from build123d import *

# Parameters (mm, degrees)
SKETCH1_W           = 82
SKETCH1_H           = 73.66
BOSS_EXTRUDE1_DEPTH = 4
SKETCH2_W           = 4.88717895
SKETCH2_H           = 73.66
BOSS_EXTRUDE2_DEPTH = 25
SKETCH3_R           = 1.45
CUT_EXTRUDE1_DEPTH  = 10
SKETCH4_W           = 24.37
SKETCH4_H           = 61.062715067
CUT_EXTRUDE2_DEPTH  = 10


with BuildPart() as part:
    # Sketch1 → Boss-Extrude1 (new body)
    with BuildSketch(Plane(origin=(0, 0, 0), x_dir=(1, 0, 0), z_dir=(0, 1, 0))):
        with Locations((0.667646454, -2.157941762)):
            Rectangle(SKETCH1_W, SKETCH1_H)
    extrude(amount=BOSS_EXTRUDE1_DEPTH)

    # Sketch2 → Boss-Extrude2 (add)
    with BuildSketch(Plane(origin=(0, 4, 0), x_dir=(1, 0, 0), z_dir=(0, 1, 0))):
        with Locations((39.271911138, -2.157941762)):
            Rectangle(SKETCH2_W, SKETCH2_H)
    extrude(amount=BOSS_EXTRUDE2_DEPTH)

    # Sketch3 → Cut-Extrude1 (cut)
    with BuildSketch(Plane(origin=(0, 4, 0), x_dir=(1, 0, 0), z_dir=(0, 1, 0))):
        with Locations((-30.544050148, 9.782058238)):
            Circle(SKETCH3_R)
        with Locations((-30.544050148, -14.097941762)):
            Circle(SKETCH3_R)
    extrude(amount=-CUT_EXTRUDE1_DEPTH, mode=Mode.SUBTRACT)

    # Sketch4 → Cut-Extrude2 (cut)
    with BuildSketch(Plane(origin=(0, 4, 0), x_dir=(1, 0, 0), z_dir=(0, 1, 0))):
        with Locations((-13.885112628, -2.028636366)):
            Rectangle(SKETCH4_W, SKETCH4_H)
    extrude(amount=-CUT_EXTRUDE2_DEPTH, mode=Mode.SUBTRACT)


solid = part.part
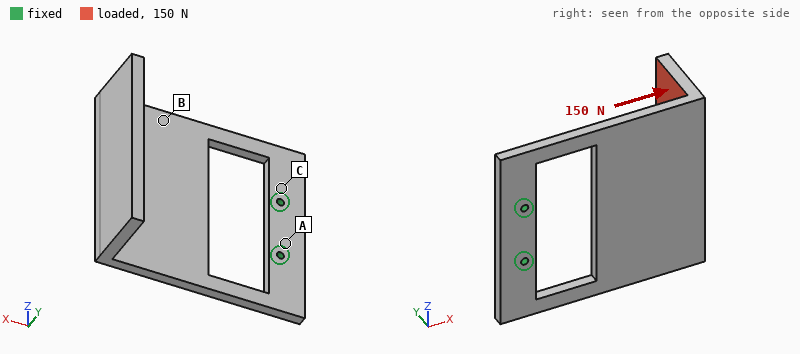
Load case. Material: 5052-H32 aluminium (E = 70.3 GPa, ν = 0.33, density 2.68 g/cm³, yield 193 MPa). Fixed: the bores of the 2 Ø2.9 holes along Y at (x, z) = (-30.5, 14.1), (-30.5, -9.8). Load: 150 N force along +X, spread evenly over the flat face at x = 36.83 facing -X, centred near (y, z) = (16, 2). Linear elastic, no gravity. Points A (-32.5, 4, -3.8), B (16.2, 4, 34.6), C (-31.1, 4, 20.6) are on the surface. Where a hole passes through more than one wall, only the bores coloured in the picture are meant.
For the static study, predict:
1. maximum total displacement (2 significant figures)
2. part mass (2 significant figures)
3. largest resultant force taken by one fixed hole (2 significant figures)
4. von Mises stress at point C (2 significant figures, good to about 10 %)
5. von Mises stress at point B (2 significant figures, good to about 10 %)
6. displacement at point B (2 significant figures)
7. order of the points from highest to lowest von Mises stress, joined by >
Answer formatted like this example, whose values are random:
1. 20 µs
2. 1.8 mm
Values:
1. 1.3 mm
2. 73 g
3. 120 N
4. 32 MPa
5. 16 MPa
6. 0.61 mm
7. C > B > A
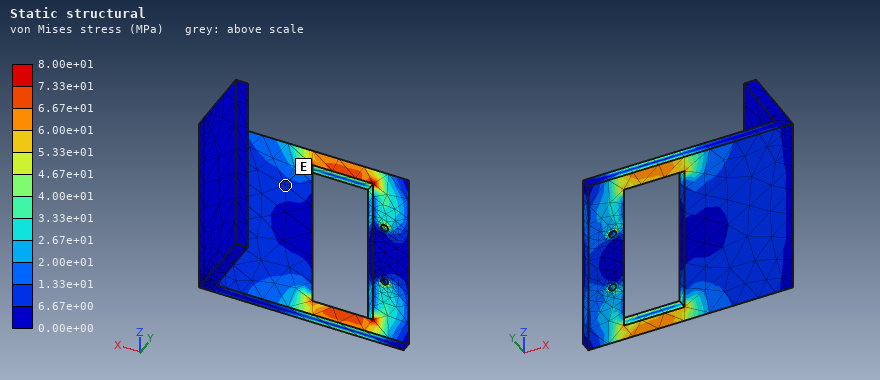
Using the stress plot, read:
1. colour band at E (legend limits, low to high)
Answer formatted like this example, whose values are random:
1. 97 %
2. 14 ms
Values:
1. 6.67e+00 to 1.33e+01 MPa
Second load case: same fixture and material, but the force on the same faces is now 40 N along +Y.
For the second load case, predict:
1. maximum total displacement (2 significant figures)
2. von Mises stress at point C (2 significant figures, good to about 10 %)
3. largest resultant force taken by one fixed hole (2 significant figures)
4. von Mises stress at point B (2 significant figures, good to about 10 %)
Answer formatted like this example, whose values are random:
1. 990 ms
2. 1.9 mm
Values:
1. 1.2 mm
2. 37 MPa
3. 20 N
4. 6.6 MPa
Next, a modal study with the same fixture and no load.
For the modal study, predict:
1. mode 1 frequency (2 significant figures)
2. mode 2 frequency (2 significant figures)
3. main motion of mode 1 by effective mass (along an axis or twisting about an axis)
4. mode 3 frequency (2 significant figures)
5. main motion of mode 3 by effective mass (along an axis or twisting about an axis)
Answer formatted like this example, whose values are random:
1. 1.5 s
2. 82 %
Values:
1. 140 Hz
2. 570 Hz
3. along Y
4. 940 Hz
5. along Z
